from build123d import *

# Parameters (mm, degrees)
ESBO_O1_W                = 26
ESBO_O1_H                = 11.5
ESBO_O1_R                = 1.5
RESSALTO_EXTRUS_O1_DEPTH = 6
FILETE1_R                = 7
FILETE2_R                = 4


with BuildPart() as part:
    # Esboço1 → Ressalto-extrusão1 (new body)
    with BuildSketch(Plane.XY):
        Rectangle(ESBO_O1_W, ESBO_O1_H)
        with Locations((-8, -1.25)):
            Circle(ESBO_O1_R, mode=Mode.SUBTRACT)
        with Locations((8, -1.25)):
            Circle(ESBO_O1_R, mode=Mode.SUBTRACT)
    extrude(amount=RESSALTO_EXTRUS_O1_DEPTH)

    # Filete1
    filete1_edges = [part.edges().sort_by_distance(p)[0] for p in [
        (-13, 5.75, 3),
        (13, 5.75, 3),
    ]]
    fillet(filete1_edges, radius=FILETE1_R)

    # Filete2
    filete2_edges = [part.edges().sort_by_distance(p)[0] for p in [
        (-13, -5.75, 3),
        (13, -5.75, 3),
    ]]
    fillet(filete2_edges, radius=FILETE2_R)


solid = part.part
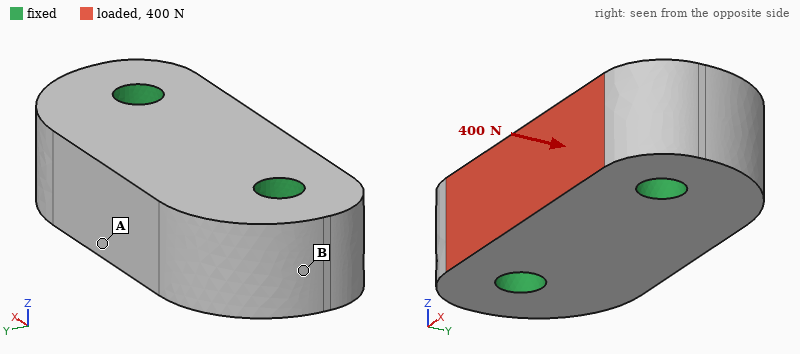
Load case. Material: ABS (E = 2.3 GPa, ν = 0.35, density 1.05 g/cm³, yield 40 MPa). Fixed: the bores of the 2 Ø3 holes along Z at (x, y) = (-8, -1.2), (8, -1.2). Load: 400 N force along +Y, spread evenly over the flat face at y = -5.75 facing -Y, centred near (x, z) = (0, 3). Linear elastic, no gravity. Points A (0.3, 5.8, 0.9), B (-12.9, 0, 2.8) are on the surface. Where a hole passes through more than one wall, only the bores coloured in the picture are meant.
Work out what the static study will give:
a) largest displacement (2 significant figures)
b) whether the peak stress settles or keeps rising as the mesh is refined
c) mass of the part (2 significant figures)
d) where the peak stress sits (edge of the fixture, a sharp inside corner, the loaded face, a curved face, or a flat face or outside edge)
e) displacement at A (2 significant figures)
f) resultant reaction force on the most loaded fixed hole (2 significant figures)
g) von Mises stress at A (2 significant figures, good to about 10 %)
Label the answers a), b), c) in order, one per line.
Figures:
a) 23 µm
b) keeps rising
c) 1.6 g
d) edge of the fixture
e) 13 µm
f) 200 N
g) 3.7 MPa
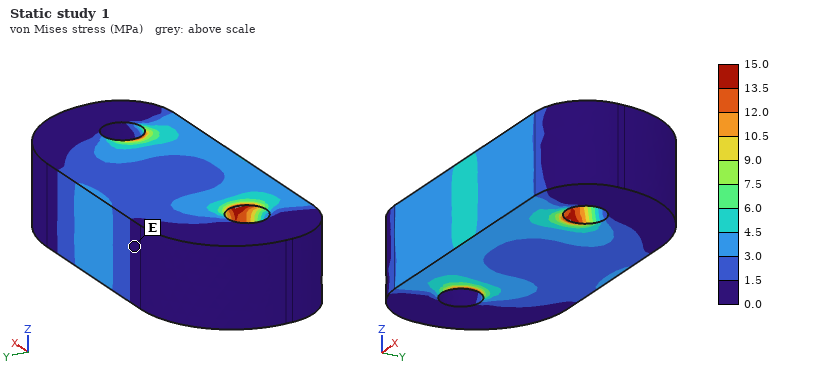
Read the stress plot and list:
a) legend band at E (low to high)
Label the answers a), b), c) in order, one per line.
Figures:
a) 0.0 to 1.5 MPa
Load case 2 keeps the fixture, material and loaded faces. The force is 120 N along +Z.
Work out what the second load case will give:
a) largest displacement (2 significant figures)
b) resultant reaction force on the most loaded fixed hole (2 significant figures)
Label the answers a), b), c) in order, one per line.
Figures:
a) 26 µm
b) 60 N
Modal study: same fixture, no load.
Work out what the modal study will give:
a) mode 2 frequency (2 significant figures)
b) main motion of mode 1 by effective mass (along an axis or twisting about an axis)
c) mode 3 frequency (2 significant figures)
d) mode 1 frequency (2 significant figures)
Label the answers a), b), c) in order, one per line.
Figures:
a) 23 kHz
b) along Z
c) 23 kHz
d) 17 kHz
